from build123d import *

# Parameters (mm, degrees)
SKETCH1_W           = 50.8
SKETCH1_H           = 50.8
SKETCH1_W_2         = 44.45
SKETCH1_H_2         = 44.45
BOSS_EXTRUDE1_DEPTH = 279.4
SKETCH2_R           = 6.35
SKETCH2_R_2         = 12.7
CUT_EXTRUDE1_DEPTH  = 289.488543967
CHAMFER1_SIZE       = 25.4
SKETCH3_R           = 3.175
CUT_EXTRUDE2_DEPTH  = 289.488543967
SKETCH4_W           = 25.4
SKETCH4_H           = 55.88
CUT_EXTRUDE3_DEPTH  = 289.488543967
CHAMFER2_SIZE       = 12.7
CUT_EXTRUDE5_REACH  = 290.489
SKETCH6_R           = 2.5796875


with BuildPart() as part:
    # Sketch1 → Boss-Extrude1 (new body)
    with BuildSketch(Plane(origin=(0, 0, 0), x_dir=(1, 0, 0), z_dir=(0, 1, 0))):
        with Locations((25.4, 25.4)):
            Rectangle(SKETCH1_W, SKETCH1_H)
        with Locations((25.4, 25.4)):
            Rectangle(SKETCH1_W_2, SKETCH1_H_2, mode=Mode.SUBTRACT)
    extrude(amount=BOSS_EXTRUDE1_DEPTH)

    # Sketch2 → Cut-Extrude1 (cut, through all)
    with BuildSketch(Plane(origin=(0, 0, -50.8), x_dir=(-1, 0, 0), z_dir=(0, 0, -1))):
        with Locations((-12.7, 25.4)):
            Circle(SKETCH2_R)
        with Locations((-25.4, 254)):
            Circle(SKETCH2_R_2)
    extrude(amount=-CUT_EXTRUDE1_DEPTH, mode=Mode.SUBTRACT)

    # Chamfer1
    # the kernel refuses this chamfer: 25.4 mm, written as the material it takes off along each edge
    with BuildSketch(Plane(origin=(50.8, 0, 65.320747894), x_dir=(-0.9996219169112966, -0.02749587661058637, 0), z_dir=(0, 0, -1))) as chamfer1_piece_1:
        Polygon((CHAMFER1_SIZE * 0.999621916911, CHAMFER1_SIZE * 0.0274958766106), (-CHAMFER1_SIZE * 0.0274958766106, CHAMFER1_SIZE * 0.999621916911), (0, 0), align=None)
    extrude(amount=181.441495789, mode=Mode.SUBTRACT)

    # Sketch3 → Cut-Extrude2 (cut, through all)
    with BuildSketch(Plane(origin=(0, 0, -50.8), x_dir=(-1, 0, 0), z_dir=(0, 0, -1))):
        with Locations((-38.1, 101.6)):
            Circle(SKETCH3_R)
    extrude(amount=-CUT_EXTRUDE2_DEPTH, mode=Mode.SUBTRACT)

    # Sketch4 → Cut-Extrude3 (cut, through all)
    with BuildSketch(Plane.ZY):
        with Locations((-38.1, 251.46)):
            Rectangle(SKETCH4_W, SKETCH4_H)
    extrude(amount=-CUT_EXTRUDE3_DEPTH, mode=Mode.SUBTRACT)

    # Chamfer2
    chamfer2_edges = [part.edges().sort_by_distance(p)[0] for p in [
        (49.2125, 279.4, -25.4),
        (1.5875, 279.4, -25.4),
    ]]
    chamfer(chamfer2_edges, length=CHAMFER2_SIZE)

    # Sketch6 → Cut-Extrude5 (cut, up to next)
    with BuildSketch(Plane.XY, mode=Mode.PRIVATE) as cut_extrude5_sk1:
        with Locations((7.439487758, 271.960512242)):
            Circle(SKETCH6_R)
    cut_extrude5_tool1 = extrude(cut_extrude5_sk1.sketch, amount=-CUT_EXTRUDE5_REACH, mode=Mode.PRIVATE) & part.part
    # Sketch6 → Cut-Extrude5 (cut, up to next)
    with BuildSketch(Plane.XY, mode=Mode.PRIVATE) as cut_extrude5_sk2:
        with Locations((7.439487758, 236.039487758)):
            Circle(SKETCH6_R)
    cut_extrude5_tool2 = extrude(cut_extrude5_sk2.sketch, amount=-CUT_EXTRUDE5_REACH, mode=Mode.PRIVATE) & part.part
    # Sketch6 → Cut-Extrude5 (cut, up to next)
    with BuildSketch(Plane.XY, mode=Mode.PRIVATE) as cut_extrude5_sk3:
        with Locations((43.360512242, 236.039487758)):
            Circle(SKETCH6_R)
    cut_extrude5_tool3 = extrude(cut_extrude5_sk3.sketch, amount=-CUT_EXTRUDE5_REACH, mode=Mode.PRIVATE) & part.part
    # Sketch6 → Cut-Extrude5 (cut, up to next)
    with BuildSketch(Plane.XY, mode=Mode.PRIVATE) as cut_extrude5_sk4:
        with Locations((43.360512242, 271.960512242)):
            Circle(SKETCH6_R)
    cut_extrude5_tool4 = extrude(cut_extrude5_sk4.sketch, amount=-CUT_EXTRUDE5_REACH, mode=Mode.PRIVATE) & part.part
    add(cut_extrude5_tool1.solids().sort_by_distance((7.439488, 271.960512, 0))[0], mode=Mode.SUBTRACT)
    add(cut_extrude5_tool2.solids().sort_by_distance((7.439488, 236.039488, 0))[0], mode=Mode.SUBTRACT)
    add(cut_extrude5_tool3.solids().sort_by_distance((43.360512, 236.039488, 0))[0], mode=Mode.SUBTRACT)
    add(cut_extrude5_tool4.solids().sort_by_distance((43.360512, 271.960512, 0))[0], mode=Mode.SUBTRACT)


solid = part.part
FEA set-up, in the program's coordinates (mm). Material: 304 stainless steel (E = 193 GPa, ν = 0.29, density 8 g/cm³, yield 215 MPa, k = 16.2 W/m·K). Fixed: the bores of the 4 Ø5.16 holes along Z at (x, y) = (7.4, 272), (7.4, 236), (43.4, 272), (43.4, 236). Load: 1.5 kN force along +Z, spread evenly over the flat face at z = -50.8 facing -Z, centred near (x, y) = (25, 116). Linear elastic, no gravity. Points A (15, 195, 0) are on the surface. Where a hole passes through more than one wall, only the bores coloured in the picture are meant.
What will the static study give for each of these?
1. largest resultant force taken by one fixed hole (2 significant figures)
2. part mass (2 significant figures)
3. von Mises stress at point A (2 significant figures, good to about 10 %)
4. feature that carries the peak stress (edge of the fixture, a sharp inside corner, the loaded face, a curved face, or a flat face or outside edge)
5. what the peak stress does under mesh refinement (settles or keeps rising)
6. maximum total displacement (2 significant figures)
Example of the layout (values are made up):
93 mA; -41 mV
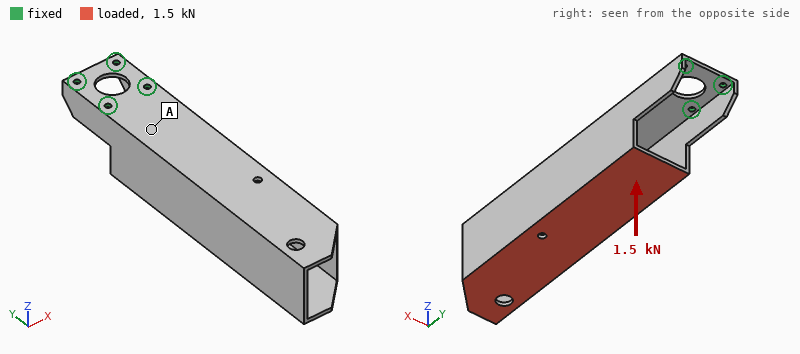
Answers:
3.7 kN; 1.1 kg; 22 MPa; edge of the fixture; keeps rising; 0.74 mm
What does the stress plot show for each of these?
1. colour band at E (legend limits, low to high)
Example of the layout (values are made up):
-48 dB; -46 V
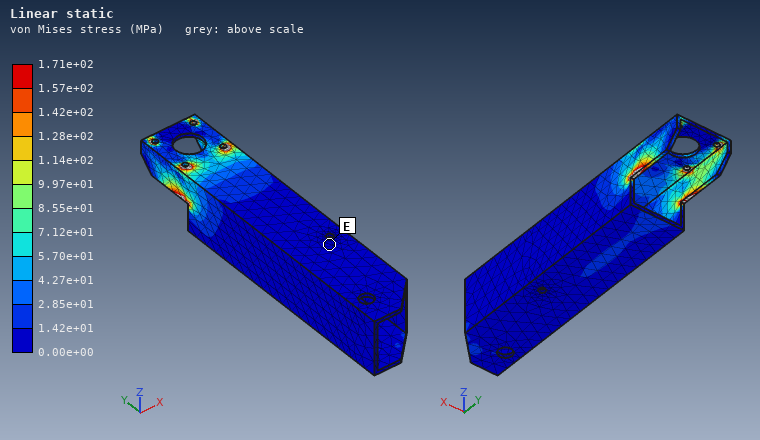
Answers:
0.00e+00 to 1.42e+01 MPa
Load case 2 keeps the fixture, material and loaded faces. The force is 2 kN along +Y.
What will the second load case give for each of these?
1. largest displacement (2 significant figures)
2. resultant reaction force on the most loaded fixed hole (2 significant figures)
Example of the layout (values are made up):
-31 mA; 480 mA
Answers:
0.37 mm; 1.8 kN
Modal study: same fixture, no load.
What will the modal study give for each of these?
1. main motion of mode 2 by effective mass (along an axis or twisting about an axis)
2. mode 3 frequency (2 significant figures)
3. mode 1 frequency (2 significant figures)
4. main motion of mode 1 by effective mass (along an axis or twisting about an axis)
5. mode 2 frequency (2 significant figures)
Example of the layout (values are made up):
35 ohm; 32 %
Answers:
along X; 770 Hz; 280 Hz; along Z; 520 Hz
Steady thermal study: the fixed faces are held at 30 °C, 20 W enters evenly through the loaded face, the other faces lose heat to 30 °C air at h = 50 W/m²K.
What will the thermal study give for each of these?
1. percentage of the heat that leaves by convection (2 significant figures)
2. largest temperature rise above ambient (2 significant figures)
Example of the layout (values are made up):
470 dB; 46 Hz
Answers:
99 %; 18 K
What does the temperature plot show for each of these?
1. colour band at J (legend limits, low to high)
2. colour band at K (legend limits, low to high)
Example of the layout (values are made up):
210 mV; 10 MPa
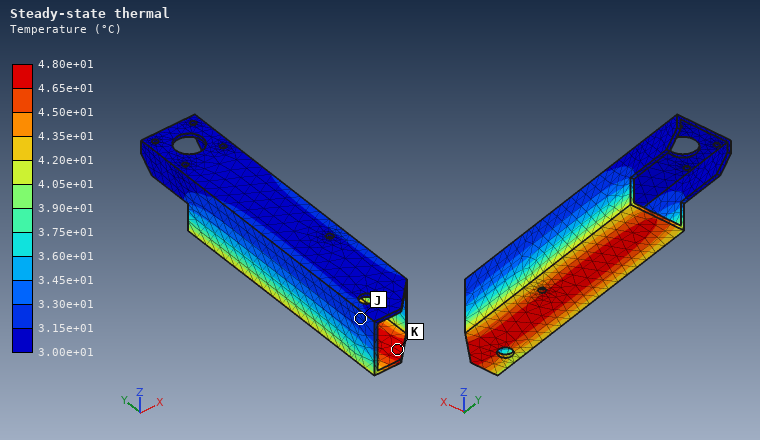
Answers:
3.15e+01 to 3.30e+01 °C; 4.65e+01 to 4.80e+01 °C
